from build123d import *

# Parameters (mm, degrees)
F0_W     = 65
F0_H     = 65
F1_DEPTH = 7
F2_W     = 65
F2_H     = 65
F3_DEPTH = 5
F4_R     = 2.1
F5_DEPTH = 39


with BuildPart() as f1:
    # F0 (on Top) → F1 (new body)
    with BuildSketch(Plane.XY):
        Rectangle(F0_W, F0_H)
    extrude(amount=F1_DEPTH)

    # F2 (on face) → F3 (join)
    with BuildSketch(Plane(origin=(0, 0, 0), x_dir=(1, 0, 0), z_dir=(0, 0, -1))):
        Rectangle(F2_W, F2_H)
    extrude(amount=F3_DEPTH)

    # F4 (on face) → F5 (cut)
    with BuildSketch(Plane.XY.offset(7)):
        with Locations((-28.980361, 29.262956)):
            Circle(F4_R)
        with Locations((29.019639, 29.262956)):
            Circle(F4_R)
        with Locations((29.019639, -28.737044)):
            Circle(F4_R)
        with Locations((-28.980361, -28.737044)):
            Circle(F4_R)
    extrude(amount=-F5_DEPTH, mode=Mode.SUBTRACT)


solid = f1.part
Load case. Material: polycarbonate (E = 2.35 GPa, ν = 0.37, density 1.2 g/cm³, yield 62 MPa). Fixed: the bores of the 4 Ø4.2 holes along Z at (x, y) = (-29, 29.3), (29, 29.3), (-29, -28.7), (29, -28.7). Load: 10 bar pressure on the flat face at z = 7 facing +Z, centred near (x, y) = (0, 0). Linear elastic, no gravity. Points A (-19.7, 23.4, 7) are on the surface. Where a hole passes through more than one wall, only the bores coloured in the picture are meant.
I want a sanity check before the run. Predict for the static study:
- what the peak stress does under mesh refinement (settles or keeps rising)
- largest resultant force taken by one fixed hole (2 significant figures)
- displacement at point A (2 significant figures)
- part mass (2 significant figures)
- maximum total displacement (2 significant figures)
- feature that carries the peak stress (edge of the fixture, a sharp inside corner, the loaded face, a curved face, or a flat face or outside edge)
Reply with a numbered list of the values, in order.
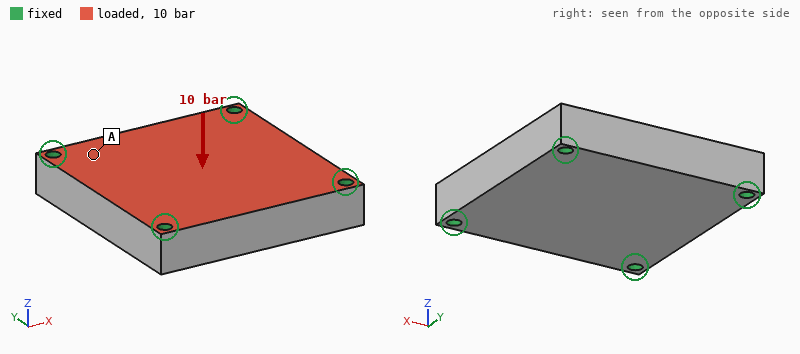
1. keeps rising
2. 1.1 kN
3. 0.15 mm
4. 60 g
5. 0.34 mm
6. edge of the fixture
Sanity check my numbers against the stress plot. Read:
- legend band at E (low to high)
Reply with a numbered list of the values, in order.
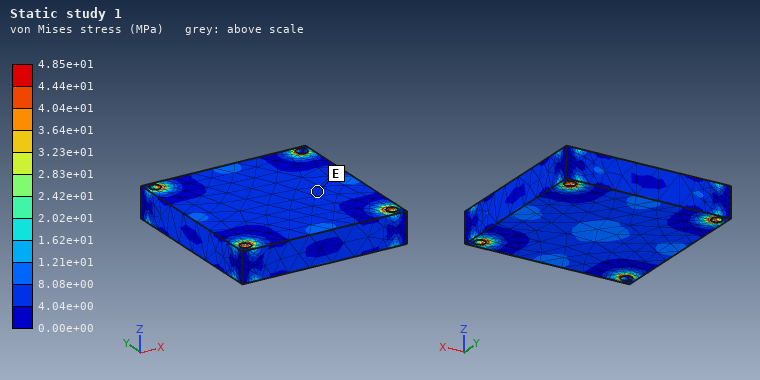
1. 4.04e+00 to 8.08e+00 MPa
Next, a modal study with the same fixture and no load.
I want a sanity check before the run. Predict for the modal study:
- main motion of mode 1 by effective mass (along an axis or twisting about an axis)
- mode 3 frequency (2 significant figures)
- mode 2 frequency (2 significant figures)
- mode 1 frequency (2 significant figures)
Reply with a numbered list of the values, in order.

1. along Z
2. 4200 Hz
3. 4200 Hz
4. 2600 Hz
